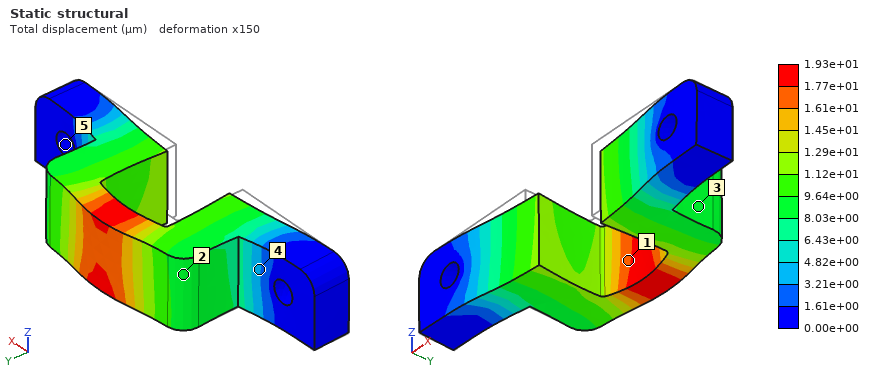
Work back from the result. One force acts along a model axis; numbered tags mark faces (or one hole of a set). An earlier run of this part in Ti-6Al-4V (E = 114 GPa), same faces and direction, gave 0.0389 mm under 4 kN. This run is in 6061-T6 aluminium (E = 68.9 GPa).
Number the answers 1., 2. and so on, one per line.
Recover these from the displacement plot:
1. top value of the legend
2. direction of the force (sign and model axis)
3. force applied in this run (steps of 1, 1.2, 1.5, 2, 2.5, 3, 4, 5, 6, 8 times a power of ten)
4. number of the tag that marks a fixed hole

1. 1.93e+01 µm
2. +Y
3. 1.2 kN
4. 5
